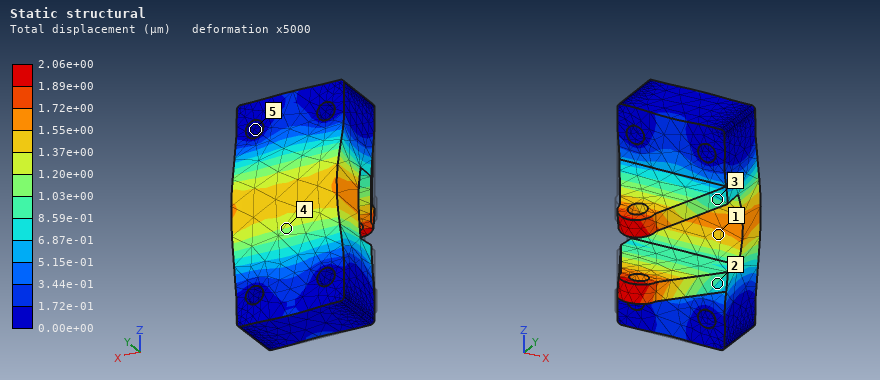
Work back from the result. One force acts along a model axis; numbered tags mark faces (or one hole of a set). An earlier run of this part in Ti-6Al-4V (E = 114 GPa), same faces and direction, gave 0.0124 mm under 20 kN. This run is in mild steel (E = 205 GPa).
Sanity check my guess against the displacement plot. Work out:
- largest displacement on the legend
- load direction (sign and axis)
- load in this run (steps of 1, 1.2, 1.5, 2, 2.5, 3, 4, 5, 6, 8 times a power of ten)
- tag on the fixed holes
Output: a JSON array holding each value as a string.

["2.06e+00 µm", "+Y", "6 kN", "5"]
